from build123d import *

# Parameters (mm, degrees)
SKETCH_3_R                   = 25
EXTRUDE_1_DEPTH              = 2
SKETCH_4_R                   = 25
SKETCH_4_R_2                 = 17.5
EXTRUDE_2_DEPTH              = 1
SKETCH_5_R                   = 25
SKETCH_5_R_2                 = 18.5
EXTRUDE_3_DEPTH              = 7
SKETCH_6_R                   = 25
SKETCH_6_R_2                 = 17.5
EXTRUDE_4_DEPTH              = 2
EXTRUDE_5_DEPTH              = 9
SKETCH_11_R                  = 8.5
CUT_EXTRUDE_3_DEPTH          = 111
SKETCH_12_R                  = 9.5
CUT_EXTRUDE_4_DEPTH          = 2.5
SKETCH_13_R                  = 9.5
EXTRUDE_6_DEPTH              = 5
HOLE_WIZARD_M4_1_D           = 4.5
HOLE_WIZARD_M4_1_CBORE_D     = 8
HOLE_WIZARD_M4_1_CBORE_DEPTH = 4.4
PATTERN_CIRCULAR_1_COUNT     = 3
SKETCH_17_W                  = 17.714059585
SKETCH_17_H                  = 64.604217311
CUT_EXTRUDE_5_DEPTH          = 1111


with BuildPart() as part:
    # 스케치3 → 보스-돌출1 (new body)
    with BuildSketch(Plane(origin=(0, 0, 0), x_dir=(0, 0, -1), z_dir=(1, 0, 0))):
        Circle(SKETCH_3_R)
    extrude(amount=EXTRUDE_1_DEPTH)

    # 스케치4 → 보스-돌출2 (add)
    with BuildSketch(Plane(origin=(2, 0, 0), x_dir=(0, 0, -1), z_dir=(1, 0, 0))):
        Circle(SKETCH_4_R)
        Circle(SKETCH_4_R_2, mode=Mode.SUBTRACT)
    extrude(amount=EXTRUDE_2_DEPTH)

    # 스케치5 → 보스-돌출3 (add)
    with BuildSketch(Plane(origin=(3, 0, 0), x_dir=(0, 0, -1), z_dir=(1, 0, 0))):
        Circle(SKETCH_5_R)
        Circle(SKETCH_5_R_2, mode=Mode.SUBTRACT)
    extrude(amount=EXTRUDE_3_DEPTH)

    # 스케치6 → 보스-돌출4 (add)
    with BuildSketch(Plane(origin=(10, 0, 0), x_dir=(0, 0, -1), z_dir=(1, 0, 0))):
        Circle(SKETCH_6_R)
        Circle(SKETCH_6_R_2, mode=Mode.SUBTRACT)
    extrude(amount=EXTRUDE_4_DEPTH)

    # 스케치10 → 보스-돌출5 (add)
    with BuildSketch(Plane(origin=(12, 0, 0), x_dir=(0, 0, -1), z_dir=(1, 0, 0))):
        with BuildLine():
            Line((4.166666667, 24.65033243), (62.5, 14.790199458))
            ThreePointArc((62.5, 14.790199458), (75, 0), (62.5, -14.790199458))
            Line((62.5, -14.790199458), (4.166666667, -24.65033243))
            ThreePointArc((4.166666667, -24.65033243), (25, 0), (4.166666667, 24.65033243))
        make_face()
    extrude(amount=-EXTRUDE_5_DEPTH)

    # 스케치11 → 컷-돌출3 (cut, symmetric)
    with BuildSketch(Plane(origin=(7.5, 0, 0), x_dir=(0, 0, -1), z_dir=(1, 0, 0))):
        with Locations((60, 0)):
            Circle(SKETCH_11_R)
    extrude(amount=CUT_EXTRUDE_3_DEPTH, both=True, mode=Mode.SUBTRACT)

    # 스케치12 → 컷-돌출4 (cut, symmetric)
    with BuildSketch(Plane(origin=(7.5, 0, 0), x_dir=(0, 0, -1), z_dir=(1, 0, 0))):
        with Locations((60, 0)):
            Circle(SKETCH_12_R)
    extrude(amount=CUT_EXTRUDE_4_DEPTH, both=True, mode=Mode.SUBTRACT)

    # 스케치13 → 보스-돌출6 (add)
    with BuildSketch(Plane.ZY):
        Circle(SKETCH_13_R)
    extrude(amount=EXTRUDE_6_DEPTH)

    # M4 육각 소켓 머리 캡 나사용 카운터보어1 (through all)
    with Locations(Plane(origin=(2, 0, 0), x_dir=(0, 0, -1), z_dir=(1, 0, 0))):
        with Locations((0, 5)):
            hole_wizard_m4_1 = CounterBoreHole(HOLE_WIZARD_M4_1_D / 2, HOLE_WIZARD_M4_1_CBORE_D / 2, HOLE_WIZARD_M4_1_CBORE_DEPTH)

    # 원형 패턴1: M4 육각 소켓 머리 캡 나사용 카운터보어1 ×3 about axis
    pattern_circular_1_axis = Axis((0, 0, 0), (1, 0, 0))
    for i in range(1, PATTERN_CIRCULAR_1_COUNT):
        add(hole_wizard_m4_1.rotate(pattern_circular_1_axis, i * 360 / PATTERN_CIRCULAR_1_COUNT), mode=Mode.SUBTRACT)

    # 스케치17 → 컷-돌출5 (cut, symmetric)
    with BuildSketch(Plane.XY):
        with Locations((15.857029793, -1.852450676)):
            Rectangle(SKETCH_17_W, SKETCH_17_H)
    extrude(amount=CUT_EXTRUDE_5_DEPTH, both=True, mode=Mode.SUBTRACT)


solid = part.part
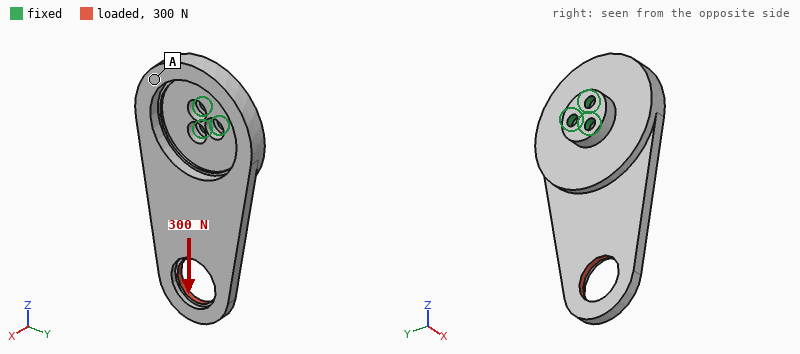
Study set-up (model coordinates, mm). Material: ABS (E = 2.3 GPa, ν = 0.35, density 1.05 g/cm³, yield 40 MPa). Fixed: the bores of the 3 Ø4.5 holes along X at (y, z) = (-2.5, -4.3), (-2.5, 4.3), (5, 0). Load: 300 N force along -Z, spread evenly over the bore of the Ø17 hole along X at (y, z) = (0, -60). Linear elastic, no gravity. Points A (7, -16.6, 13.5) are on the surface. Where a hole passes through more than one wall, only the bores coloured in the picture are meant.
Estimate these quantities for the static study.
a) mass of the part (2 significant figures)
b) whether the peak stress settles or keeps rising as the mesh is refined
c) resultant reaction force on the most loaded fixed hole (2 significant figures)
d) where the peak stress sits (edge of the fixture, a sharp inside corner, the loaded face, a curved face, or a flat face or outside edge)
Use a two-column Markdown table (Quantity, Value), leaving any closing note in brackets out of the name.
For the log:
| Quantity | Value |
|---|---|
| mass of the part | 16 g |
| whether the peak stress settles or keeps rising as the mesh is refined | keeps rising |
| resultant reaction force on the most loaded fixed hole | 190 N |
| where the peak stress sits | edge of the fixture |
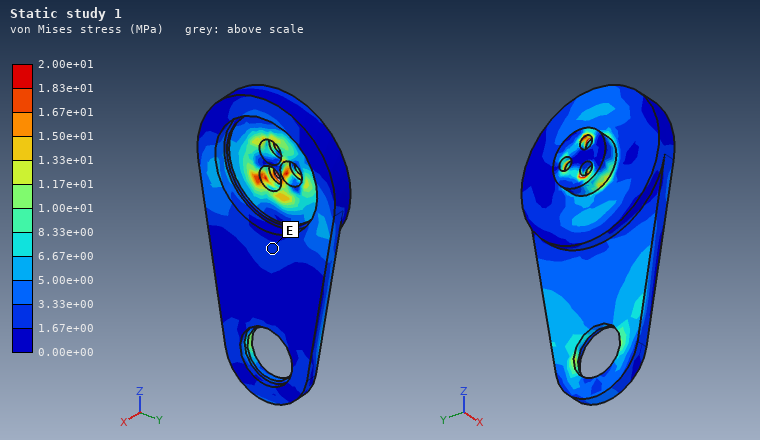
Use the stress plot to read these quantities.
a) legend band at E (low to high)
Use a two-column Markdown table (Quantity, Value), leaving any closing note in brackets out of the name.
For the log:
| Quantity | Value |
|---|---|
| legend band at E | 1.67e+00 to 3.33e+00 MPa |
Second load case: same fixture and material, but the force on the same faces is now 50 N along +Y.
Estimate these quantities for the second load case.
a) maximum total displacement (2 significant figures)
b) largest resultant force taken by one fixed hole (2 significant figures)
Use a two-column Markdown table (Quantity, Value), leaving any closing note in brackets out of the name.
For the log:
| Quantity | Value |
|---|---|
| maximum total displacement | 0.50 mm |
| largest resultant force taken by one fixed hole | 170 N |
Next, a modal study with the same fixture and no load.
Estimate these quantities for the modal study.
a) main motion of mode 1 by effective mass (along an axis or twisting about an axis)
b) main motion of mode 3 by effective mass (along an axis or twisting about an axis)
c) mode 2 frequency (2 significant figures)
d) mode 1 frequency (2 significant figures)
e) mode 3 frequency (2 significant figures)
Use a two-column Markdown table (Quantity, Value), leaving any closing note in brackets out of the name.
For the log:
| Quantity | Value |
|---|---|
| main motion of mode 1 by effective mass | along X |
| main motion of mode 3 by effective mass | along Y |
| mode 2 frequency | 720 Hz |
| mode 1 frequency | 260 Hz |
| mode 3 frequency | 910 Hz |
